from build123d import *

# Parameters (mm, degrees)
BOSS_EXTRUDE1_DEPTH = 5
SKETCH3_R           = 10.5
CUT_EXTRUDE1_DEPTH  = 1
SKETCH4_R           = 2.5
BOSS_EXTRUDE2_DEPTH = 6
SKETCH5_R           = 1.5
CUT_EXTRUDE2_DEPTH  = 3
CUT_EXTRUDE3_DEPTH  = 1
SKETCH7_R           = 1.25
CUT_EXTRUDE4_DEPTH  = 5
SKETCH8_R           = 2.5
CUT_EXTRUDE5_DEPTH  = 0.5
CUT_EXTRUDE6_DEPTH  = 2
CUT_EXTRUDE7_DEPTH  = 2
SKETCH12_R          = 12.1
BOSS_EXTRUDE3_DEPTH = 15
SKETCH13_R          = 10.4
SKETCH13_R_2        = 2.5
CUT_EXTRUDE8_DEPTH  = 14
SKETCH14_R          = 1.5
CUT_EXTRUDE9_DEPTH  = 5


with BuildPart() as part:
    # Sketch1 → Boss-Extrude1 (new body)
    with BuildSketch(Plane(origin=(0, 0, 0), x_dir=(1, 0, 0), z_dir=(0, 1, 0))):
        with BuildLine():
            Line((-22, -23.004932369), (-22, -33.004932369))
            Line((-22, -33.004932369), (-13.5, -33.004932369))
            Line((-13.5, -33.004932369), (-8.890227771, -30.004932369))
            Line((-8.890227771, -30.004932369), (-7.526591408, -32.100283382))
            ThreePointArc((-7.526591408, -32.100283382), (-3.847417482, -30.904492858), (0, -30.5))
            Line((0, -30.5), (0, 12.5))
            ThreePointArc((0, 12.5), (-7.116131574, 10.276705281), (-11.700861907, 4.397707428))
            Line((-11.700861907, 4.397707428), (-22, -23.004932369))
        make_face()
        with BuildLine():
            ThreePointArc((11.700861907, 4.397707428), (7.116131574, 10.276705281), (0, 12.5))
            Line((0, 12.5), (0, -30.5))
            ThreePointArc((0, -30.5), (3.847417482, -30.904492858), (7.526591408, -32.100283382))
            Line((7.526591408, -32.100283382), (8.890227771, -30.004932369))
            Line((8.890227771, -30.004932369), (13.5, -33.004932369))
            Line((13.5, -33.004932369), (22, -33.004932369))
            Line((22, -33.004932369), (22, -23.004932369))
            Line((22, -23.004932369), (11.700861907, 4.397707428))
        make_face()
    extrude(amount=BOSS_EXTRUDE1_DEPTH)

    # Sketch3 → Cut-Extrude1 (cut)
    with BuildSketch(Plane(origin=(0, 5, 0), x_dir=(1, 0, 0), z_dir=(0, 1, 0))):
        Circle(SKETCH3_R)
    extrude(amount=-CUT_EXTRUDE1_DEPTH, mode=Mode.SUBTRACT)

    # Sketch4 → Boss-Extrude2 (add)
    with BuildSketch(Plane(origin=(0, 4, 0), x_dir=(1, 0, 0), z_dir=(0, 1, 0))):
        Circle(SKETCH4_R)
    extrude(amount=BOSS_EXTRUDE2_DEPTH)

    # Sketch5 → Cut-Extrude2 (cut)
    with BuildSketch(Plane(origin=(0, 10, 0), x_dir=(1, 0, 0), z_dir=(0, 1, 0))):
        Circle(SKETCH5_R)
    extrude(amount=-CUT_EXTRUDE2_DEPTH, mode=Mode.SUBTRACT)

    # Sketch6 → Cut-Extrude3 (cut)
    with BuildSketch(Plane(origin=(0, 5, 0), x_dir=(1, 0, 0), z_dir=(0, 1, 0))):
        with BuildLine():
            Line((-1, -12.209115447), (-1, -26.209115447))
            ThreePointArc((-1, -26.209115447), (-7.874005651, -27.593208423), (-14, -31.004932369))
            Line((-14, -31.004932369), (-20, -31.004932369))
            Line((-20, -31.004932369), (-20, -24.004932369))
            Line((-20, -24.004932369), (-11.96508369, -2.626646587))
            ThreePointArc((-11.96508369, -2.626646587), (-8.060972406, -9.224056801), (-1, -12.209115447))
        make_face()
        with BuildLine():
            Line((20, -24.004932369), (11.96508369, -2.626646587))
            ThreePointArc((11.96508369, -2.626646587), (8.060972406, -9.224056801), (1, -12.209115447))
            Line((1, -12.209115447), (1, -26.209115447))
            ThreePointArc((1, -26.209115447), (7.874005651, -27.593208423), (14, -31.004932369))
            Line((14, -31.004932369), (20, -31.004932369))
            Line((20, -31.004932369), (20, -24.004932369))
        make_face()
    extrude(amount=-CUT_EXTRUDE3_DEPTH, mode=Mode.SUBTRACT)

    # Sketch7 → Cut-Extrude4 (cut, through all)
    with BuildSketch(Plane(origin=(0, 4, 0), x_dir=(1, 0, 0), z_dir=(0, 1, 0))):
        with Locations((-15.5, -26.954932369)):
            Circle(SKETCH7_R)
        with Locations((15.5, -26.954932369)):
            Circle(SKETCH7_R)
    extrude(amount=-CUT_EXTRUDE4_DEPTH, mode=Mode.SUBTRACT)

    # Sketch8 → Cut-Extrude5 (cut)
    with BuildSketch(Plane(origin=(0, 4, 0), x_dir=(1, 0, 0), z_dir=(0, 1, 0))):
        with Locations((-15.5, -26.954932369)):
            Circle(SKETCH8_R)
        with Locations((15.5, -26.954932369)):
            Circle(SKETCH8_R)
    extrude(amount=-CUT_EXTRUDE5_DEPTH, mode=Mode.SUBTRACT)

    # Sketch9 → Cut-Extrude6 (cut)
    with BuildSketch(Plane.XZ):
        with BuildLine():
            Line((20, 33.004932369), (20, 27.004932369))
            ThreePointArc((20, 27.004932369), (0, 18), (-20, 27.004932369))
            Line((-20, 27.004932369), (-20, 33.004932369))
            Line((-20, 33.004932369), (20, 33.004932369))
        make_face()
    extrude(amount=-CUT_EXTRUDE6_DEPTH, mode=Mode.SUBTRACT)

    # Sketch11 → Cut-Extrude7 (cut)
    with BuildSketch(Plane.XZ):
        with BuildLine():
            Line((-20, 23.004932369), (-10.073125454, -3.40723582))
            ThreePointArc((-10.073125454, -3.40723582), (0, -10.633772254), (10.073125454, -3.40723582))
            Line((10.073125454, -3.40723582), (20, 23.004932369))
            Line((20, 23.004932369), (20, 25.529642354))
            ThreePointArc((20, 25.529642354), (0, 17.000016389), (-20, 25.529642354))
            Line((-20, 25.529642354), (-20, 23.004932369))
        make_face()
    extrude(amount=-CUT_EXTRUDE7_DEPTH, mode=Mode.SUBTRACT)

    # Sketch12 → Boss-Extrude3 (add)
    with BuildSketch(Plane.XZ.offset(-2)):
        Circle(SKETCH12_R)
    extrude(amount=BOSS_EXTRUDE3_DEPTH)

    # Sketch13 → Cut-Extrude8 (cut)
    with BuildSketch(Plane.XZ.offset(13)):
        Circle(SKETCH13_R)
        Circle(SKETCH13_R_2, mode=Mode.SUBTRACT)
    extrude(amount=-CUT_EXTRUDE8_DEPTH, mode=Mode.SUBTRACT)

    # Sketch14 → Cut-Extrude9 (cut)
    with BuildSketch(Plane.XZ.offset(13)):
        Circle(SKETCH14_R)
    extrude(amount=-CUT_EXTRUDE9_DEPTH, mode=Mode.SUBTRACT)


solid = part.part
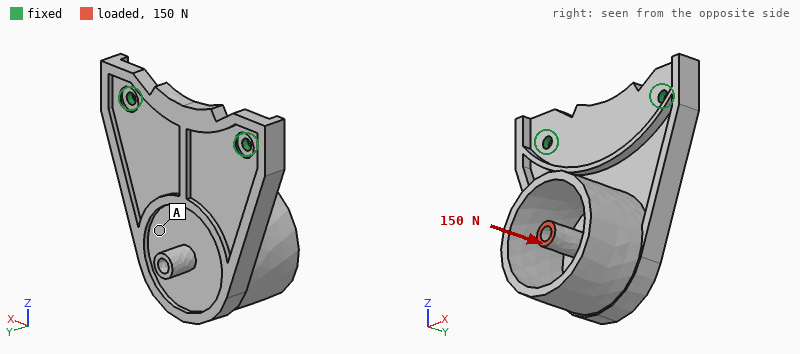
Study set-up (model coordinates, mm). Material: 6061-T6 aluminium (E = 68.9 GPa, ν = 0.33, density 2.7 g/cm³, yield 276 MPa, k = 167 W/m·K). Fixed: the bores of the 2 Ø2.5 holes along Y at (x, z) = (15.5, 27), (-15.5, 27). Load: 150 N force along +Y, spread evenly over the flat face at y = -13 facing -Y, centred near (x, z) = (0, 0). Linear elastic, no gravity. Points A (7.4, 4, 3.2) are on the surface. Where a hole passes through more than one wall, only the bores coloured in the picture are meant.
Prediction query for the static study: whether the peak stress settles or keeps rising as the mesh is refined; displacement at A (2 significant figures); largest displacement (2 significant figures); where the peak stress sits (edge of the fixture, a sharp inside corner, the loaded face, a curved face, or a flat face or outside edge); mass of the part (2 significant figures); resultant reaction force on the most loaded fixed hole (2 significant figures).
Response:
keeps rising
0.33 mm
0.66 mm
edge of the fixture
17 g
78 N
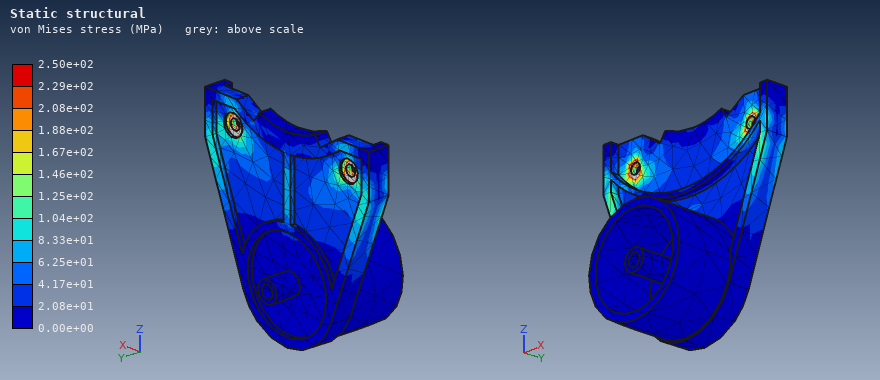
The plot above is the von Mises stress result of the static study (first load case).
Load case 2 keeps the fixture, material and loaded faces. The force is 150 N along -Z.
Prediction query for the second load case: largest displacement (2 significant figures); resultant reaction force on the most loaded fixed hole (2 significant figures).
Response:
0.51 mm
76 N
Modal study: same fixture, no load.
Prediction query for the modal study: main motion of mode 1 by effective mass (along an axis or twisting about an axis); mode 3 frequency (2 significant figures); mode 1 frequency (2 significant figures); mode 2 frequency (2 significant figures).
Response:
along Y
5200 Hz
880 Hz
3400 Hz
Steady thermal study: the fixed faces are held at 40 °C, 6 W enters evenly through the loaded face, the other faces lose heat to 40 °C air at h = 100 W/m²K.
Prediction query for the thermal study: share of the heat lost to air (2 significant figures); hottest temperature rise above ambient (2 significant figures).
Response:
54 %
39 K
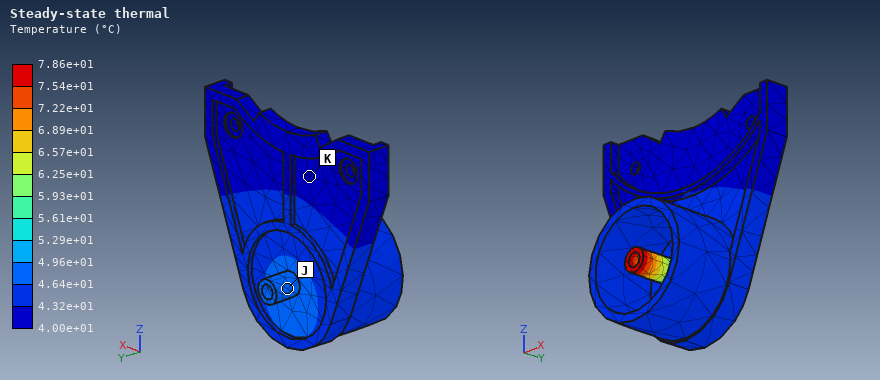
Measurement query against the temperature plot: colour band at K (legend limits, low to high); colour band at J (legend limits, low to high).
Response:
4.00e+01 to 4.32e+01 °C
4.64e+01 to 4.96e+01 °C
